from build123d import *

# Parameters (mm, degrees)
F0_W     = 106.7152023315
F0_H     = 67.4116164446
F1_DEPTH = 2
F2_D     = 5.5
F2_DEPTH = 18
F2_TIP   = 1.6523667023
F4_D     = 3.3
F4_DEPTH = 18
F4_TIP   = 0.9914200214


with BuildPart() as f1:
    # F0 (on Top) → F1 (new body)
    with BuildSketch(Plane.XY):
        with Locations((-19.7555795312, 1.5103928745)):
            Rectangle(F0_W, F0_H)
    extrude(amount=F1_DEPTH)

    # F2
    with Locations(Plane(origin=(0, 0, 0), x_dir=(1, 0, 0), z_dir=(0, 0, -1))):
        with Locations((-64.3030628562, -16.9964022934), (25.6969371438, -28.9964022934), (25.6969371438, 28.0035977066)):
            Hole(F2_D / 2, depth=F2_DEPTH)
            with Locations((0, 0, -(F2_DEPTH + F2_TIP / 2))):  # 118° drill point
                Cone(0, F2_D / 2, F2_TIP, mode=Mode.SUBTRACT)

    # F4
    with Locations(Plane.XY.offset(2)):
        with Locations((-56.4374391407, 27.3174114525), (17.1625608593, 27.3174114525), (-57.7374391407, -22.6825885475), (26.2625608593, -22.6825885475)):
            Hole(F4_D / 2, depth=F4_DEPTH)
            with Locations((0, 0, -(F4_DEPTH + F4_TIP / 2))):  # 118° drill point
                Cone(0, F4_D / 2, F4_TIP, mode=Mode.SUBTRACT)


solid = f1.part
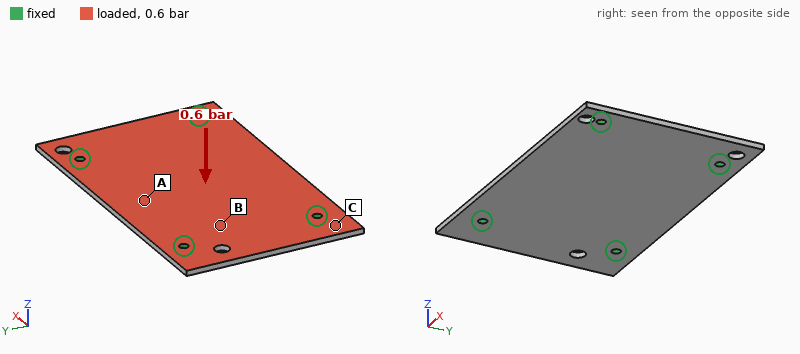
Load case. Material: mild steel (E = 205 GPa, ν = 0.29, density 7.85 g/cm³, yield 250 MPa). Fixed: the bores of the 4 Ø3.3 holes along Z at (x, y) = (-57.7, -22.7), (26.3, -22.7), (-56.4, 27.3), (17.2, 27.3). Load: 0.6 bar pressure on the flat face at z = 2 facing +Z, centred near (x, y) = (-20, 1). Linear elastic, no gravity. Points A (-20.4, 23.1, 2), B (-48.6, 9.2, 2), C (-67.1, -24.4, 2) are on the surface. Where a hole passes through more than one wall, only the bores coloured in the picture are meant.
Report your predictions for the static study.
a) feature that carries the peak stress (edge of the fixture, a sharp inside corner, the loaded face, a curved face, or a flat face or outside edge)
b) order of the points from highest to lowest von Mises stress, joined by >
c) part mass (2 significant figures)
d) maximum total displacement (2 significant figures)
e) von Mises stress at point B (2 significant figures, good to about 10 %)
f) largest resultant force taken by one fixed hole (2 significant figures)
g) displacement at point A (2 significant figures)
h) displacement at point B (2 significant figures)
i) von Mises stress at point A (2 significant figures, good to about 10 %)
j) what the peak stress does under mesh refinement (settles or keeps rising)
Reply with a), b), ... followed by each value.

a) edge of the fixture
b) A > B > C
c) 110 g
d) 68 µm
e) 16 MPa
f) 120 N
g) 46 µm
h) 21 µm
i) 23 MPa
j) keeps rising
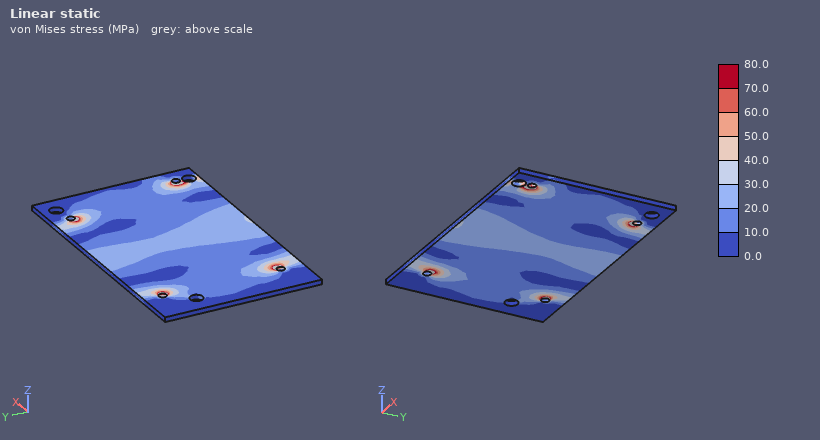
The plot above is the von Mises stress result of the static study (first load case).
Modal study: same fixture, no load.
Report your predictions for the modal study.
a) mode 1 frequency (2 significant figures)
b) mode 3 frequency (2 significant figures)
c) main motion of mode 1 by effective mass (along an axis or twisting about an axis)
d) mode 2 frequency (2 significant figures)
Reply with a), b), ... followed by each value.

a) 1400 Hz
b) 3300 Hz
c) along Z
d) 2200 Hz
